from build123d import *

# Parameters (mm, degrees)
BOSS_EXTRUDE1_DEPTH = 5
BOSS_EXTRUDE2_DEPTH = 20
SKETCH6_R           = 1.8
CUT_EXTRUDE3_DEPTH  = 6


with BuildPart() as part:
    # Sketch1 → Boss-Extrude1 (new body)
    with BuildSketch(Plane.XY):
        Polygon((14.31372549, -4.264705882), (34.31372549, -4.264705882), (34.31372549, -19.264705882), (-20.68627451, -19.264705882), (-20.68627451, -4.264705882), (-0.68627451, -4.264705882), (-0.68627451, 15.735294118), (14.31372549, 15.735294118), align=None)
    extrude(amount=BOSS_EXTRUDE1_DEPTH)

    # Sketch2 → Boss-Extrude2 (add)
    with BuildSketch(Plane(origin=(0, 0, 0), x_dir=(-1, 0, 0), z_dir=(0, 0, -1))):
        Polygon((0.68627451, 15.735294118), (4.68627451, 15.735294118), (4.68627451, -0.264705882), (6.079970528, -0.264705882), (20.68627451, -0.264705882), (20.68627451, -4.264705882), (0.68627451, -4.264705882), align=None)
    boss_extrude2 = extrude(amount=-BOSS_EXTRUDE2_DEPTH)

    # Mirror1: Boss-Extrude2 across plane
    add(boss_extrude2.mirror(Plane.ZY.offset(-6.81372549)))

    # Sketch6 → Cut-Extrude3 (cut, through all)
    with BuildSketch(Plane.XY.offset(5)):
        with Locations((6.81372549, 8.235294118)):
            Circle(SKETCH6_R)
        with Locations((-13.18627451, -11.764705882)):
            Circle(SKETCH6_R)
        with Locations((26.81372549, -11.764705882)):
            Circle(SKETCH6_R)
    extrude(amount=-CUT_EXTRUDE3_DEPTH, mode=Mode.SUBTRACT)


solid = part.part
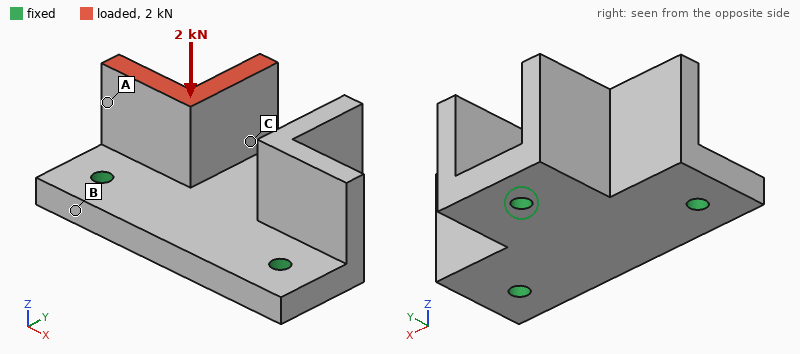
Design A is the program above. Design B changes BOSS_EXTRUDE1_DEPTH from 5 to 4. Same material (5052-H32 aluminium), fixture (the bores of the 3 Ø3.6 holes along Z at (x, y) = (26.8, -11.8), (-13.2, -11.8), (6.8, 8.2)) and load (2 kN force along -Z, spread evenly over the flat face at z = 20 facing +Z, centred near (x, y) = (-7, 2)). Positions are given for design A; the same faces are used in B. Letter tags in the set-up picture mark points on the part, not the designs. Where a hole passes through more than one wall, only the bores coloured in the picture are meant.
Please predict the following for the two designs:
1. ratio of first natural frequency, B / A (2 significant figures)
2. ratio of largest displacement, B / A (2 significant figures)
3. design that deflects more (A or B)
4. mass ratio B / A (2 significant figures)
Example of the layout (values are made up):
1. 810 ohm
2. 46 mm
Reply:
1. 0.77
2. 1.6
3. B
4. 0.90
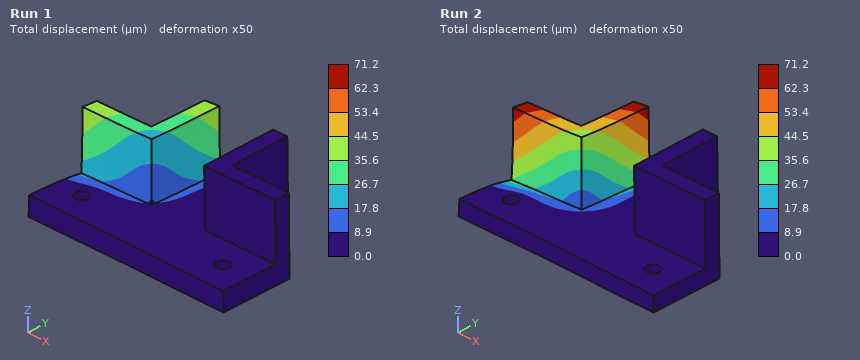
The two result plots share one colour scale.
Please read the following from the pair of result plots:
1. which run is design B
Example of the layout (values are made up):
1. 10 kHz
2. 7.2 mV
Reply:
1. Run 2
